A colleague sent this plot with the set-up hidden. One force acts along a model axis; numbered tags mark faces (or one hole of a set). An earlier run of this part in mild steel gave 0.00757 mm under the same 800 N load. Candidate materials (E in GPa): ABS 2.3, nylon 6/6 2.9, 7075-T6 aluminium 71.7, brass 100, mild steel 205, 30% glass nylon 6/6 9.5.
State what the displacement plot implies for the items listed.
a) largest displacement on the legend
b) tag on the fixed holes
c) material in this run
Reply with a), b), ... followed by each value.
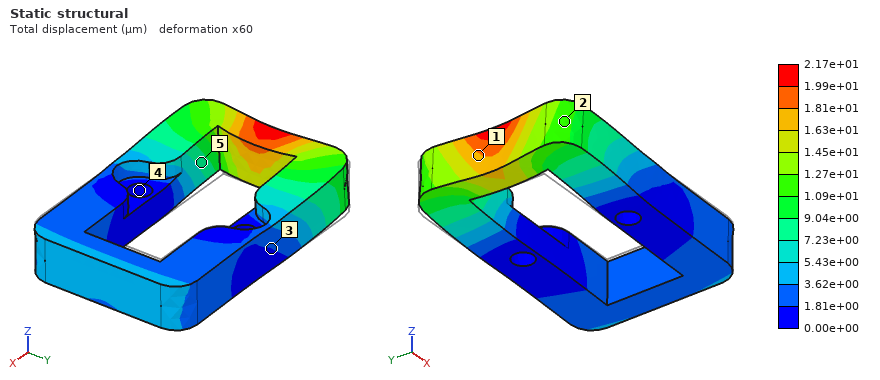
a) 2.17e+01 µm
b) 4
c) 7075-T6 aluminium
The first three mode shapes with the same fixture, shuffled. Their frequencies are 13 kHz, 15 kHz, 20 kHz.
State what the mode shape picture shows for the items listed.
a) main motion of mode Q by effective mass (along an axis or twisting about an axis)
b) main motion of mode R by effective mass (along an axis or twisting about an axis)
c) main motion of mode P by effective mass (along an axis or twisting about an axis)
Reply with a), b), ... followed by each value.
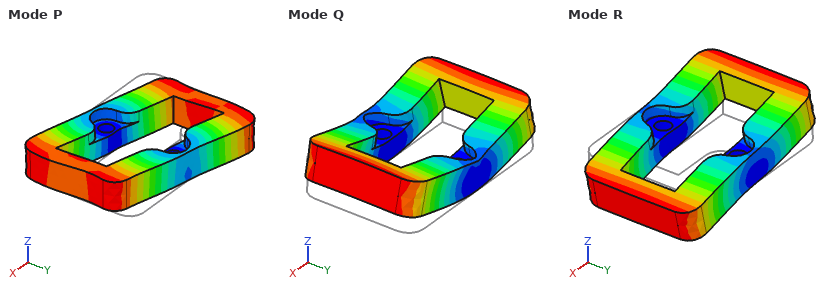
a) along Z
b) twisting about Y
c) twisting about Z
